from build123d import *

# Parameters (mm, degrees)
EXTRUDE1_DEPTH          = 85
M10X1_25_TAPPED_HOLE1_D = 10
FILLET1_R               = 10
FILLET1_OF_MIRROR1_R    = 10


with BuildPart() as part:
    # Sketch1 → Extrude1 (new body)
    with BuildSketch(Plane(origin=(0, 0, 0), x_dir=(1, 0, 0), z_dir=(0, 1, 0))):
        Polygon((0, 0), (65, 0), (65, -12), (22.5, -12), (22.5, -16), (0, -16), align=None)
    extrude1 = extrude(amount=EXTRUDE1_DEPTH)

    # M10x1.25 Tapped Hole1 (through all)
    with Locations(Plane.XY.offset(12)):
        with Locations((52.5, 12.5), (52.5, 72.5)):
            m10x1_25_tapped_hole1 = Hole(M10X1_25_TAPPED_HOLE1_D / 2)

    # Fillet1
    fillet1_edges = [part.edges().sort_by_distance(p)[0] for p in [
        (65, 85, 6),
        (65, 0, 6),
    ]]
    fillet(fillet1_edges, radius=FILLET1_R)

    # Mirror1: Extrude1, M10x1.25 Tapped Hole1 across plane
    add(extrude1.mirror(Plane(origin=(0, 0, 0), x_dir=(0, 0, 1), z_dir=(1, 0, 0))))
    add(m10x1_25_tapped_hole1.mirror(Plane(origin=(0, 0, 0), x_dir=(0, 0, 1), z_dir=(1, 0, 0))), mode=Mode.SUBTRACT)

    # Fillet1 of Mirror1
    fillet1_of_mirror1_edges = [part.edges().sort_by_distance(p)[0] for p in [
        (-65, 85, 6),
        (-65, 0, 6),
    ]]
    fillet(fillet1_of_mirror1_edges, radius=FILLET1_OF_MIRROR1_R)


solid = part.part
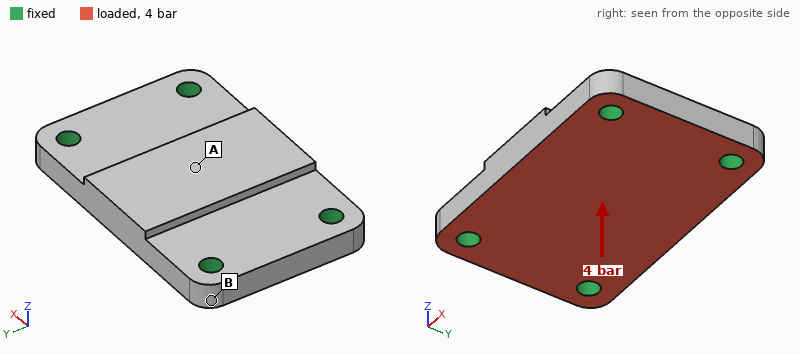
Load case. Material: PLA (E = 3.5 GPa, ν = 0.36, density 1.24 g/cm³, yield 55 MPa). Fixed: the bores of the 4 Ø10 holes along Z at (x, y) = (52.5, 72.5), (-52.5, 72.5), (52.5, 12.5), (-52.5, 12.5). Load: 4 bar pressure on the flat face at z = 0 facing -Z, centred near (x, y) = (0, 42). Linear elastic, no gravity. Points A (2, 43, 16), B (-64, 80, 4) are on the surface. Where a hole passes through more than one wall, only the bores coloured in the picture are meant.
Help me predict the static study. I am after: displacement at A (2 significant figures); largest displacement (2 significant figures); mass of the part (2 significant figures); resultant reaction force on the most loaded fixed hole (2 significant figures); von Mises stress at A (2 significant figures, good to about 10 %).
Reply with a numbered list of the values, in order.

1. 0.22 mm
2. 0.22 mm
3. 180 g
4. 1.1 kN
5. 4.6 MPa
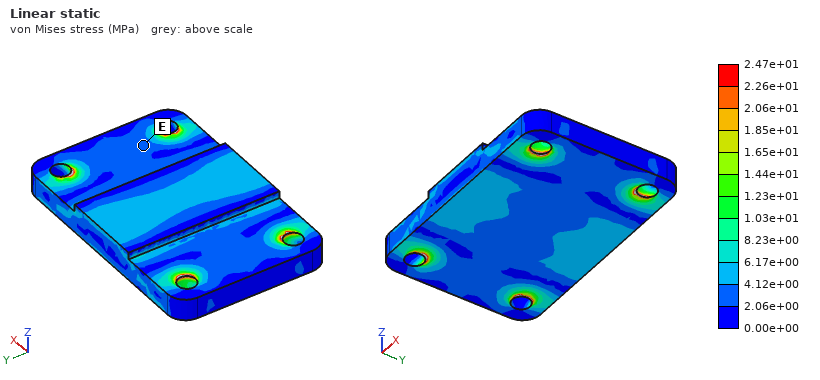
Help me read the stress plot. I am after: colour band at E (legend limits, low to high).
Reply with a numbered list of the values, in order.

1. 2.06e+00 to 4.12e+00 MPa
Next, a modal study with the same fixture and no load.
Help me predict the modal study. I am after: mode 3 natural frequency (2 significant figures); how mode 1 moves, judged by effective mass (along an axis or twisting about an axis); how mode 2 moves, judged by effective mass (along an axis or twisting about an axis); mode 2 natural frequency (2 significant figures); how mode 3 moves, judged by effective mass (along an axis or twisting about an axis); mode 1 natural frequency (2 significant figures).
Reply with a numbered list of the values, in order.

1. 3800 Hz
2. along Z
3. twisting about X
4. 2300 Hz
5. along Y
6. 1800 Hz
